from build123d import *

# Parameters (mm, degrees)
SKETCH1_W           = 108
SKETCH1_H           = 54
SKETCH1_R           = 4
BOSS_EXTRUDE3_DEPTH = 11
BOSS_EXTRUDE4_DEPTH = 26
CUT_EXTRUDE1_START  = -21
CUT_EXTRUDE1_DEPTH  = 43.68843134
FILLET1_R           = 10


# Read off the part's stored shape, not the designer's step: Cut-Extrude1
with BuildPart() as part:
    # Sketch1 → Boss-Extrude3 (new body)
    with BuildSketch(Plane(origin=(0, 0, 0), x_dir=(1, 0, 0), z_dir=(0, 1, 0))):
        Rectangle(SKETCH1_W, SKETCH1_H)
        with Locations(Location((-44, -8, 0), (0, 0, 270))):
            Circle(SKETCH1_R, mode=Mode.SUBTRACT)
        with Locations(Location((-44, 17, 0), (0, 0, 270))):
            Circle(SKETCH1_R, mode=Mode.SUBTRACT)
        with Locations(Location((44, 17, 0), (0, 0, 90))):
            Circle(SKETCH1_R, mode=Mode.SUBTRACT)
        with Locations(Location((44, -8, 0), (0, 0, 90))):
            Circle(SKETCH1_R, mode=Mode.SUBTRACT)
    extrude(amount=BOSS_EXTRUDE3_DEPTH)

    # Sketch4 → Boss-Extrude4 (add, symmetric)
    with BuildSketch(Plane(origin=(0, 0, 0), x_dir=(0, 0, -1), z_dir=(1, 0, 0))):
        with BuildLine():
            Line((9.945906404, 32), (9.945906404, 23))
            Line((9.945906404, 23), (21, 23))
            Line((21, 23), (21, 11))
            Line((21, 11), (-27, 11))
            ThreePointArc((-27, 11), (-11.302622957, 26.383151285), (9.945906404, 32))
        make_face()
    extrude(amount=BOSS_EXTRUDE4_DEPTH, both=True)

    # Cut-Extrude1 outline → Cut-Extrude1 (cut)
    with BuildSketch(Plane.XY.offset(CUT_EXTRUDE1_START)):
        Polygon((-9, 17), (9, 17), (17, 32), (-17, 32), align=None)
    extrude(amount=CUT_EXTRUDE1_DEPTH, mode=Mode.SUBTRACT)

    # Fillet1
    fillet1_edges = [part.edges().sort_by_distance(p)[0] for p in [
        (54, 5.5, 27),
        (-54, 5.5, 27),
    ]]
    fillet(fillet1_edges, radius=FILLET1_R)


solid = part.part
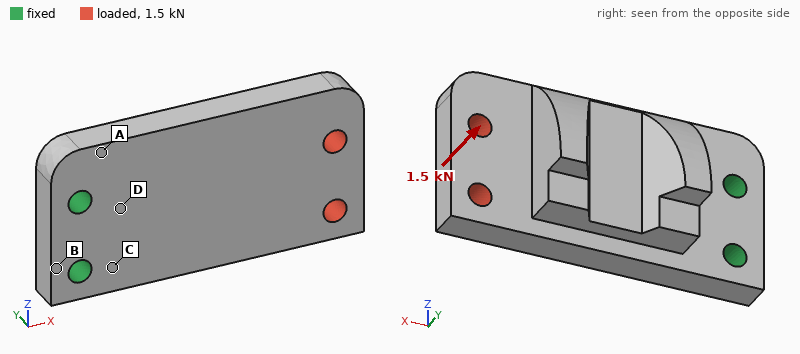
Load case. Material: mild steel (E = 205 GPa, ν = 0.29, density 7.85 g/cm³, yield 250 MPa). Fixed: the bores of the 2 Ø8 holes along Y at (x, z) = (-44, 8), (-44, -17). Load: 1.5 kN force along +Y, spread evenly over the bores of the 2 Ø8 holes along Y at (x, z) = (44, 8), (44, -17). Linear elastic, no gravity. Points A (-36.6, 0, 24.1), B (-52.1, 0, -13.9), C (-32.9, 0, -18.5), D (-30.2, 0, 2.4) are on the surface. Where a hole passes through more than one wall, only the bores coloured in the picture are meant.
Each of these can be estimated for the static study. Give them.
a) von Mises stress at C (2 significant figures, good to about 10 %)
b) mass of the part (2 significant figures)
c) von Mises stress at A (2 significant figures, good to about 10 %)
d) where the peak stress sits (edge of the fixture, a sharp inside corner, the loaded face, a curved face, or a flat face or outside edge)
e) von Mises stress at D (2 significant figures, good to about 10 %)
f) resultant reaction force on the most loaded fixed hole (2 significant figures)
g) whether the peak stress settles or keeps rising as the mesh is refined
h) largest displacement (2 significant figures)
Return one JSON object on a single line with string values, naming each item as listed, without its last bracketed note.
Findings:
{"von Mises stress at C": "110 MPa", "mass of the part": "680 g", "von Mises stress at A": "74 MPa", "where the peak stress sits": "edge of the fixture", "von Mises stress at D": "94 MPa", "resultant reaction force on the most loaded fixed hole": "790 N", "whether the peak stress settles or keeps rising as the mesh is refined": "keeps rising", "largest displacement": "0.22 mm"}
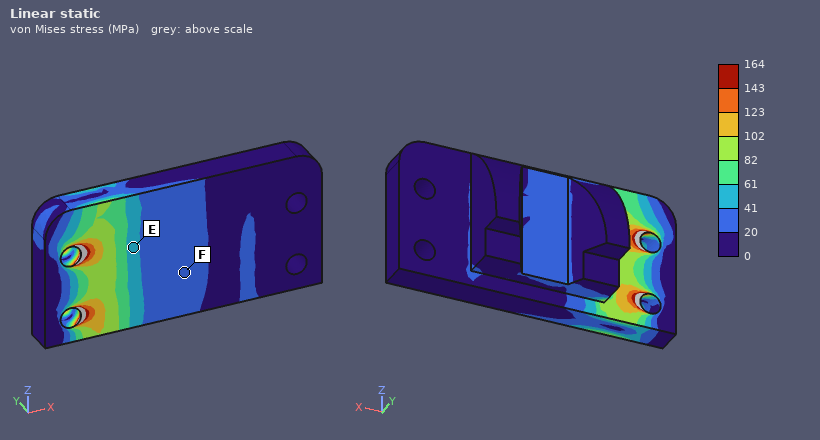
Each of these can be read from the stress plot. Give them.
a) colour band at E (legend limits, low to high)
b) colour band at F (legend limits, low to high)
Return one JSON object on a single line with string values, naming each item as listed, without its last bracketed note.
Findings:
{"colour band at E": "41 to 61 MPa", "colour band at F": "20 to 41 MPa"}
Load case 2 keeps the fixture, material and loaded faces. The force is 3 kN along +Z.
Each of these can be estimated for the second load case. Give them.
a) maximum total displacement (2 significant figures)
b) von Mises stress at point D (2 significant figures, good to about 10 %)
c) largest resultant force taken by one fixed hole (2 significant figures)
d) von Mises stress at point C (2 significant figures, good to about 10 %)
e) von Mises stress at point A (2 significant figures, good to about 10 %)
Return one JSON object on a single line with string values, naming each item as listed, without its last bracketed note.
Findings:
{"maximum total displacement": "42 µm", "von Mises stress at point D": "28 MPa", "largest resultant force taken by one fixed hole": "8.6 kN", "von Mises stress at point C": "38 MPa", "von Mises stress at point A": "15 MPa"}
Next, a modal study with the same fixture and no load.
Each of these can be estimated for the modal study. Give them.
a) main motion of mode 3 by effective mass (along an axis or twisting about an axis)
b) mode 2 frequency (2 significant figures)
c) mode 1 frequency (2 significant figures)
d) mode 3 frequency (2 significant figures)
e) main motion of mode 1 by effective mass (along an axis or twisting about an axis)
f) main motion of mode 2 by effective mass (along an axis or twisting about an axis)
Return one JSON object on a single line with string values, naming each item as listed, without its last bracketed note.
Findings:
{"main motion of mode 3 by effective mass": "twisting about X", "mode 2 frequency": "3200 Hz", "mode 1 frequency": "1000 Hz", "mode 3 frequency": "4300 Hz", "main motion of mode 1 by effective mass": "along Y", "main motion of mode 2 by effective mass": "along Z"}
